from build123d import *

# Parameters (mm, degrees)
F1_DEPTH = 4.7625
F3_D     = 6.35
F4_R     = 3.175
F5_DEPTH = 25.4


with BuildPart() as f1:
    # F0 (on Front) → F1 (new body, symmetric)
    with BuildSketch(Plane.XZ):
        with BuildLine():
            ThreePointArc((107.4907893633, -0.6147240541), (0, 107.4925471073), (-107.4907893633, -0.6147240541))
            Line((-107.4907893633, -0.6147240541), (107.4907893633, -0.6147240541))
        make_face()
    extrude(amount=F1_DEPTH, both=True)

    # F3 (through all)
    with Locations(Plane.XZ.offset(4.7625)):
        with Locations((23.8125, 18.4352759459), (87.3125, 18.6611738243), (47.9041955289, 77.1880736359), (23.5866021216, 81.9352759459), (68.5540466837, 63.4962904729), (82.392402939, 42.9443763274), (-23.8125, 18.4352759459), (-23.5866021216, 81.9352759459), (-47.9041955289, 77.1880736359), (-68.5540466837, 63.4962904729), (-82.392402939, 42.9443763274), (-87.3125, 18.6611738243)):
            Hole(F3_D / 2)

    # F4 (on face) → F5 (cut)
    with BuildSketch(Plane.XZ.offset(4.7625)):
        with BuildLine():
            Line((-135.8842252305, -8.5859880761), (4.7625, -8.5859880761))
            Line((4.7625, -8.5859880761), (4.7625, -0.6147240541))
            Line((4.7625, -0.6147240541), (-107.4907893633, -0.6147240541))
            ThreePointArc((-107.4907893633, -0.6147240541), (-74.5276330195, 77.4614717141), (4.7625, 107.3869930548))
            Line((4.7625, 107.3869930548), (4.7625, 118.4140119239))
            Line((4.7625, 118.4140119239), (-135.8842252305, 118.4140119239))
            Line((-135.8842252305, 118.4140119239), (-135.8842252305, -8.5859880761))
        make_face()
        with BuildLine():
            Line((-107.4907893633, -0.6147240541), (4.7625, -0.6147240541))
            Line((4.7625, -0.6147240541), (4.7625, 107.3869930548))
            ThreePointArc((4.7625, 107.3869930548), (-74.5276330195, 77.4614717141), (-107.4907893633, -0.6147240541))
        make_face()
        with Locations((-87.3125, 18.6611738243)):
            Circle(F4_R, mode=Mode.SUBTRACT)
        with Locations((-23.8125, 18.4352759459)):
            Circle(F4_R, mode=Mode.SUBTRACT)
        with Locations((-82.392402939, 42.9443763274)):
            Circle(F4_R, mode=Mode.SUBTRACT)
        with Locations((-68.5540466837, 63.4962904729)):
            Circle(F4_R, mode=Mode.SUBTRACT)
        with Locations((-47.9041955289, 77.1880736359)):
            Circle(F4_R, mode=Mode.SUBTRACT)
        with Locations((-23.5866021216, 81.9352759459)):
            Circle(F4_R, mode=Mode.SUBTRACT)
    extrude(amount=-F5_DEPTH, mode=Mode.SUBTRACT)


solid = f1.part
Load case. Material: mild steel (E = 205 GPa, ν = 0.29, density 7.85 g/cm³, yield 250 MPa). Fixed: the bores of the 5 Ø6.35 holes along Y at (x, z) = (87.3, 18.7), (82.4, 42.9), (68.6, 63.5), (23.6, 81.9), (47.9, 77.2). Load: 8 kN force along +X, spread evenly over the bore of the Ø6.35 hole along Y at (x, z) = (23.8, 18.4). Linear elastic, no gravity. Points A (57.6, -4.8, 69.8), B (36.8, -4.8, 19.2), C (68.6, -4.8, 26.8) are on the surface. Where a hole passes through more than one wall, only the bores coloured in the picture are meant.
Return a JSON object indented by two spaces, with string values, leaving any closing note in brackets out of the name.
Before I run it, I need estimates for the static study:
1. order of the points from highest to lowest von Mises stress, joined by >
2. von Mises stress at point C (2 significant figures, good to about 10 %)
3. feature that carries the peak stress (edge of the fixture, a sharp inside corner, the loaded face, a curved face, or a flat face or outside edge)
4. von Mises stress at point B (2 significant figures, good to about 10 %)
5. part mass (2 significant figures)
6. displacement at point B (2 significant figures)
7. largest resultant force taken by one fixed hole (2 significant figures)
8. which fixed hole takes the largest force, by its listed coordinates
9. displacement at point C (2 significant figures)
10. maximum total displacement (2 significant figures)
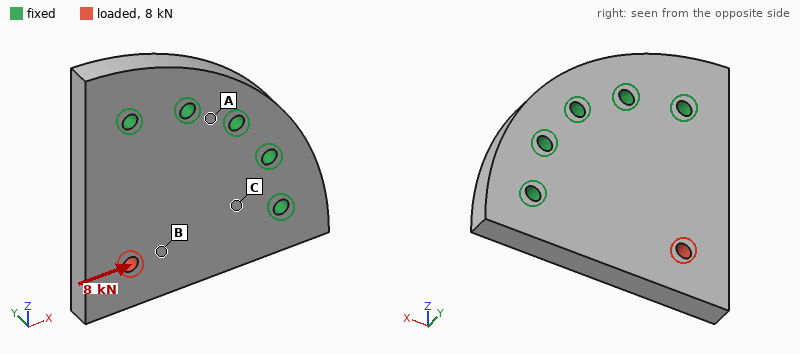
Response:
{
  "order of the points from highest to lowest von Mises stress, joined by >": "B > C > A",
  "von Mises stress at point C": "15 MPa",
  "feature that carries the peak stress": "the loaded face",
  "von Mises stress at point B": "29 MPa",
  "part mass": "630 g",
  "displacement at point B": "4.9 µm",
  "largest resultant force taken by one fixed hole": "4.5 kN",
  "which fixed hole takes the largest force, by its listed coordinates": "(87.3, 18.7)",
  "displacement at point C": "1.4 µm",
  "maximum total displacement": "7.8 µm"
}
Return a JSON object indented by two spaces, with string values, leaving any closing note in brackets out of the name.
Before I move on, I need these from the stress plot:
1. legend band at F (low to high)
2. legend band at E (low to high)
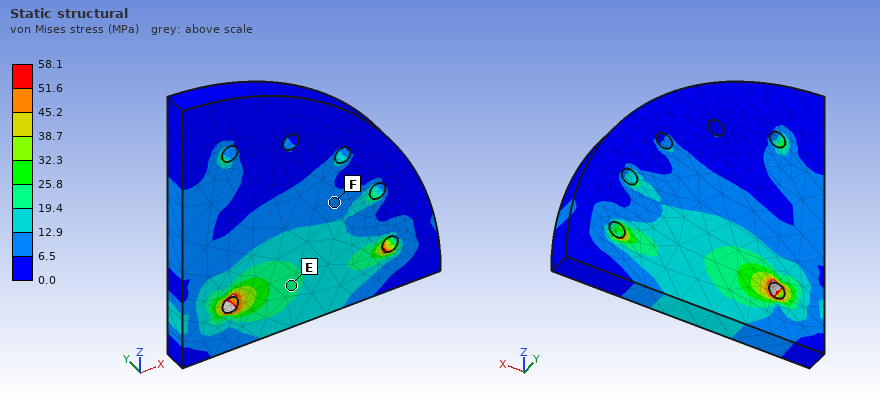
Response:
{
  "legend band at F": "6.5 to 12.9 MPa",
  "legend band at E": "19.4 to 25.8 MPa"
}
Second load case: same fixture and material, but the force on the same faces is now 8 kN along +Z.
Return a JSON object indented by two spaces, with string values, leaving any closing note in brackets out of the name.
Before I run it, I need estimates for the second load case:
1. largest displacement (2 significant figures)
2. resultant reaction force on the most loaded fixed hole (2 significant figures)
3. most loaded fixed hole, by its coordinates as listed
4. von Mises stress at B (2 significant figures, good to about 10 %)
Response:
{
  "largest displacement": "7.8 µm",
  "resultant reaction force on the most loaded fixed hole": "4.5 kN",
  "most loaded fixed hole, by its coordinates as listed": "(23.6, 81.9)",
  "von Mises stress at B": "14 MPa"
}
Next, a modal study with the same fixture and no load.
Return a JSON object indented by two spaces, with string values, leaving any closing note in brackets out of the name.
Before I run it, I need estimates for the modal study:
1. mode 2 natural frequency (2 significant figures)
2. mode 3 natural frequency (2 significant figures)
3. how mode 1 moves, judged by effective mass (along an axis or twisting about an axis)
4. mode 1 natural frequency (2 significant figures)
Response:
{
  "mode 2 natural frequency": "6900 Hz",
  "mode 3 natural frequency": "8700 Hz",
  "how mode 1 moves, judged by effective mass": "along Y",
  "mode 1 natural frequency": "2200 Hz"
}
